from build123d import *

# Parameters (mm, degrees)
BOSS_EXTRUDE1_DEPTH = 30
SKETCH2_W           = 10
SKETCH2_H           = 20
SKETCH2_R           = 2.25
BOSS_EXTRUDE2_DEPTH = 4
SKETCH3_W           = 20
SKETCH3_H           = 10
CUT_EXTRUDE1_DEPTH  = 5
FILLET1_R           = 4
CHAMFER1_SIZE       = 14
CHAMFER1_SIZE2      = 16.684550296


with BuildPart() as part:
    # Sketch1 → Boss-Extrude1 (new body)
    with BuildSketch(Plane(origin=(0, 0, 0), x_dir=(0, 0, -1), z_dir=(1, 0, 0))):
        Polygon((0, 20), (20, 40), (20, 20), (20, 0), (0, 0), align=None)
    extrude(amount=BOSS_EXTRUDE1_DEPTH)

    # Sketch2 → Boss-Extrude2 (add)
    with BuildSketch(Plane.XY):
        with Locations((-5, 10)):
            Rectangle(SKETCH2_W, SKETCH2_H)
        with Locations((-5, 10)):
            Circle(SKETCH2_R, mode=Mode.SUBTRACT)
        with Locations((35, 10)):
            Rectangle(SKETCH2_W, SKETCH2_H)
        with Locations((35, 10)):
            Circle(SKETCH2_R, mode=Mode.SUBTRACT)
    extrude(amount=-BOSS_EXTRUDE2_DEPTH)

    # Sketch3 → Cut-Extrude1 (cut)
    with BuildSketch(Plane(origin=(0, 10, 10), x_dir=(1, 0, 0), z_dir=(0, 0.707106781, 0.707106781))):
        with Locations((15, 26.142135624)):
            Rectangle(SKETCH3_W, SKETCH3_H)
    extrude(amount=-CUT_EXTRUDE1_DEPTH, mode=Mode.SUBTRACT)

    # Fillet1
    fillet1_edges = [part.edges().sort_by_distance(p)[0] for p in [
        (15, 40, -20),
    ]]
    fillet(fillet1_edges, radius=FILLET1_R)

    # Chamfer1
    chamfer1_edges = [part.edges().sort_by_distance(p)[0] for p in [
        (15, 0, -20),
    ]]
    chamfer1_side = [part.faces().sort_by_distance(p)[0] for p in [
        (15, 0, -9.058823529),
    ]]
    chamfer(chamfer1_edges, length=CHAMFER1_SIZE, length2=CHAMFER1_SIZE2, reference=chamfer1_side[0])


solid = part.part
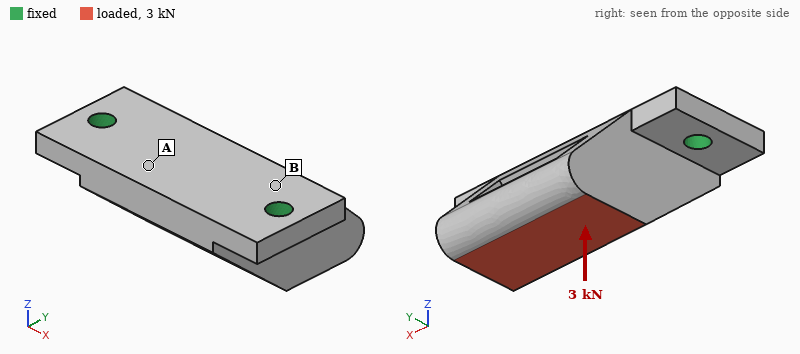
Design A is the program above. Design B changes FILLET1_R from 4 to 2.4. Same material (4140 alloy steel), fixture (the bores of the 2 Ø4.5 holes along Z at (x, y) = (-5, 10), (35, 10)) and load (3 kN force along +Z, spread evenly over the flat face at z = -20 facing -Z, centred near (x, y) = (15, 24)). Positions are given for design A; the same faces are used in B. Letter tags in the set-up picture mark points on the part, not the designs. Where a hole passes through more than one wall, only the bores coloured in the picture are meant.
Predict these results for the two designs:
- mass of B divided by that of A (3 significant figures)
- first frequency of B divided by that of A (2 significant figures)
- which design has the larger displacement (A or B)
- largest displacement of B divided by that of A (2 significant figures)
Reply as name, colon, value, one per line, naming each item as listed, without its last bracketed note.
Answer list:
mass of B divided by that of A: 1.03
first frequency of B divided by that of A: 0.94
which design has the larger displacement: B
largest displacement of B divided by that of A: 1.3
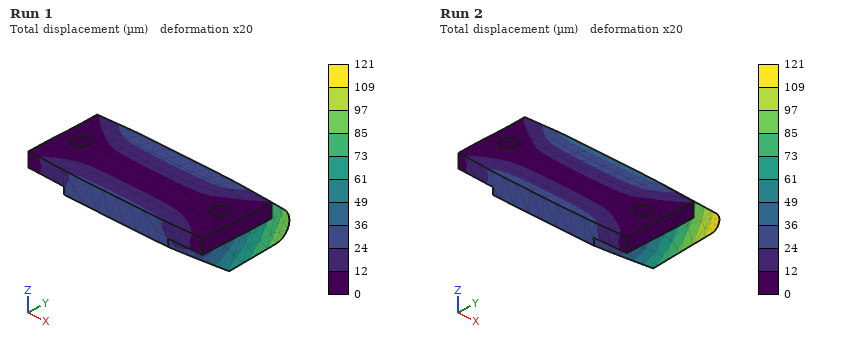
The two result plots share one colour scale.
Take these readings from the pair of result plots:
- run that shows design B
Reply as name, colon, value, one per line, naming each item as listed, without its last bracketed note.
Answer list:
run that shows design B: Run 2
